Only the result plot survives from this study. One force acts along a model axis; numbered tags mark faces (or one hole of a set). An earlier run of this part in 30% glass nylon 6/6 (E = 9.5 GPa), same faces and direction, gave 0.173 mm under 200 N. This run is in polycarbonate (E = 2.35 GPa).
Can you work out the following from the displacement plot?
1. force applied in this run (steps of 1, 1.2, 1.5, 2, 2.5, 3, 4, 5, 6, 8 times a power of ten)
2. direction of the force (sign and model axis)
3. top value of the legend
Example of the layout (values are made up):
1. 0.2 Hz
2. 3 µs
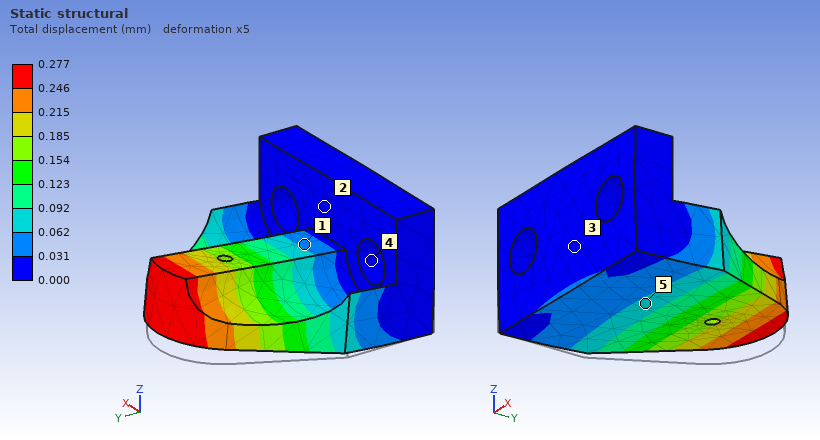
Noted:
1. 80 N
2. +Z
3. 0.277 mm
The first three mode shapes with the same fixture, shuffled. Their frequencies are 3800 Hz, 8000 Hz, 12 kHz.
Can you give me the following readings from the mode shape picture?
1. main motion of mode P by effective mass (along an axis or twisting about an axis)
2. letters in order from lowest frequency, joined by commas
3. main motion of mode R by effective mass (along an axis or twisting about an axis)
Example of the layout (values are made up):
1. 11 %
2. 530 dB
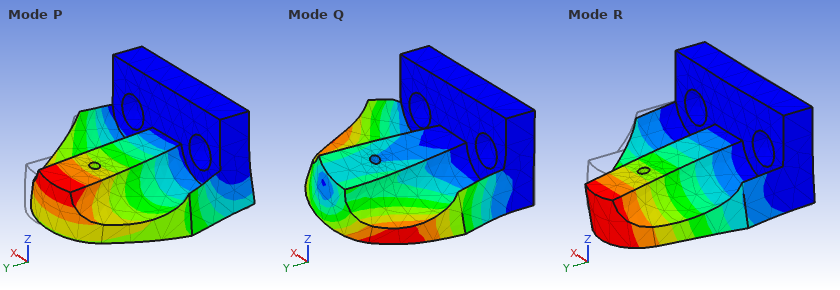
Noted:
1. along X
2. R, P, Q
3. along Z
